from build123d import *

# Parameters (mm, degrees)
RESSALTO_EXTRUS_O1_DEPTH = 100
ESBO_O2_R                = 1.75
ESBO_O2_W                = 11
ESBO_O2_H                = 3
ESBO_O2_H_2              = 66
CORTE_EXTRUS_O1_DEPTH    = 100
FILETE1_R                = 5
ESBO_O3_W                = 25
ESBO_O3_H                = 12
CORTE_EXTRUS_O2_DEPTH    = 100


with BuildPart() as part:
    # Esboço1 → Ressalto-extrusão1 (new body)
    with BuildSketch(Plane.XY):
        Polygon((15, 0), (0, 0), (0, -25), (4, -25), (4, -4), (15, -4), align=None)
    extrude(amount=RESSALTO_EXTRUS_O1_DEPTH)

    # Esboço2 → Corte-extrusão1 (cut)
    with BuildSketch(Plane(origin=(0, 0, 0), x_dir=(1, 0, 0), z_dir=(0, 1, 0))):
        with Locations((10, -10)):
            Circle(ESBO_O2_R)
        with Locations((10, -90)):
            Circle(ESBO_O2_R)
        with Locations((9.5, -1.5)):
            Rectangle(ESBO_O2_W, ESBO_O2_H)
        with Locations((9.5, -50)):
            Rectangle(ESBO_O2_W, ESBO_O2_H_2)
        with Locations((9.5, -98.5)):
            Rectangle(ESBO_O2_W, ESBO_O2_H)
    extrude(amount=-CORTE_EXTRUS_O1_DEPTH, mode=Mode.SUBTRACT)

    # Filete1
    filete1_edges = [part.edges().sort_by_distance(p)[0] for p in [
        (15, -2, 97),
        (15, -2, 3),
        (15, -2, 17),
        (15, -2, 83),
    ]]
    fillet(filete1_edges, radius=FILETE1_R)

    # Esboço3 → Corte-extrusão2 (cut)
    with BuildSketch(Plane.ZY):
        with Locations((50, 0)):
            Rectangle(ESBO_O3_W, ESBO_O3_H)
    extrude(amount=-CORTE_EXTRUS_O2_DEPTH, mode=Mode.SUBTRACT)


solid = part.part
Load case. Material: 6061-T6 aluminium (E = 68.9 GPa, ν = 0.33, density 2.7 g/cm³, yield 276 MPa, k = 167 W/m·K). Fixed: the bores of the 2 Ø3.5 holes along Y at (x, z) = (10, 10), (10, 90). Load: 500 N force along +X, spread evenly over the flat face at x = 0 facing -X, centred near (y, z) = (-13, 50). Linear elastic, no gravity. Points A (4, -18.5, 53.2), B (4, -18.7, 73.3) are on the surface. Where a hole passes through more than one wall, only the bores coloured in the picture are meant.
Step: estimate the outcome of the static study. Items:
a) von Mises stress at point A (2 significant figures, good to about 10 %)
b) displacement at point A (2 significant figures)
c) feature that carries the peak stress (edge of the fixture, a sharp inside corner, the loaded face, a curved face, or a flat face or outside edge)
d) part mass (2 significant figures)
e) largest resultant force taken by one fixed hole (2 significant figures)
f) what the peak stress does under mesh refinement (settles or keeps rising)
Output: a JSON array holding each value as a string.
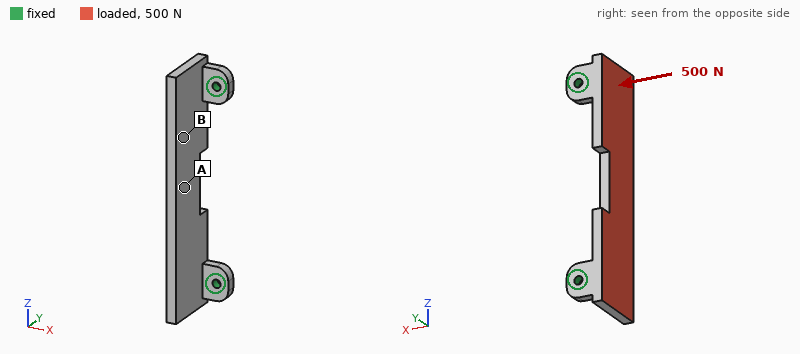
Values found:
["23 MPa", "0.16 mm", "edge of the fixture", "28 g", "270 N", "keeps rising"]
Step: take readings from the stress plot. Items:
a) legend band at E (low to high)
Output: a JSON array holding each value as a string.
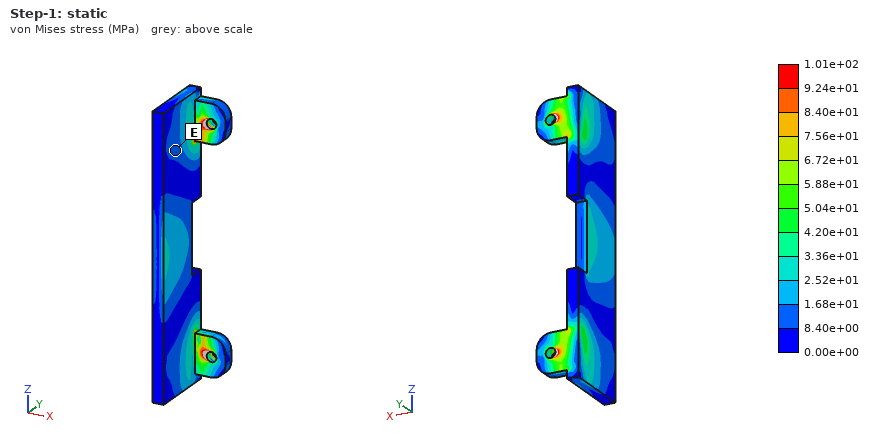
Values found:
["8.40e+00 to 1.68e+01 MPa"]
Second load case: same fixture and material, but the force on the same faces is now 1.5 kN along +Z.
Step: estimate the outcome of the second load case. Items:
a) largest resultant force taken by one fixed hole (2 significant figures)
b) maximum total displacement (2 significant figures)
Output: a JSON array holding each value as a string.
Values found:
["780 N", "28 µm"]
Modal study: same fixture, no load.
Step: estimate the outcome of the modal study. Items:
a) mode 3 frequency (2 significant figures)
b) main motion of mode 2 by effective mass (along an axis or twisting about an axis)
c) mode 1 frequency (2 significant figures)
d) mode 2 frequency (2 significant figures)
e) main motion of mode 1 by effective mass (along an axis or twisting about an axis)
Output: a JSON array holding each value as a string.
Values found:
["4400 Hz", "twisting about Y", "2000 Hz", "4000 Hz", "along X"]
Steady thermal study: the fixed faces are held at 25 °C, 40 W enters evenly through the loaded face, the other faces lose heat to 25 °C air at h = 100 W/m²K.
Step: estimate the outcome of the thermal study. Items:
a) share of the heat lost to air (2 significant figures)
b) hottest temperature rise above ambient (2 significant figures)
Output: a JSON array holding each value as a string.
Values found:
["21 %", "31 K"]
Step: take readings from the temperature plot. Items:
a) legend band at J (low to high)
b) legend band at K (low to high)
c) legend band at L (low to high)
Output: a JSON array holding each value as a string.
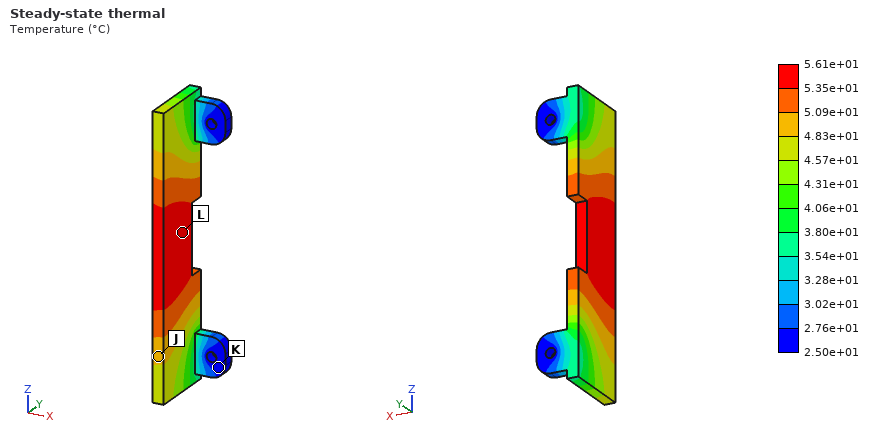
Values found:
["4.83e+01 to 5.09e+01 °C", "2.50e+01 to 2.76e+01 °C", "5.35e+01 to 5.61e+01 °C"]
